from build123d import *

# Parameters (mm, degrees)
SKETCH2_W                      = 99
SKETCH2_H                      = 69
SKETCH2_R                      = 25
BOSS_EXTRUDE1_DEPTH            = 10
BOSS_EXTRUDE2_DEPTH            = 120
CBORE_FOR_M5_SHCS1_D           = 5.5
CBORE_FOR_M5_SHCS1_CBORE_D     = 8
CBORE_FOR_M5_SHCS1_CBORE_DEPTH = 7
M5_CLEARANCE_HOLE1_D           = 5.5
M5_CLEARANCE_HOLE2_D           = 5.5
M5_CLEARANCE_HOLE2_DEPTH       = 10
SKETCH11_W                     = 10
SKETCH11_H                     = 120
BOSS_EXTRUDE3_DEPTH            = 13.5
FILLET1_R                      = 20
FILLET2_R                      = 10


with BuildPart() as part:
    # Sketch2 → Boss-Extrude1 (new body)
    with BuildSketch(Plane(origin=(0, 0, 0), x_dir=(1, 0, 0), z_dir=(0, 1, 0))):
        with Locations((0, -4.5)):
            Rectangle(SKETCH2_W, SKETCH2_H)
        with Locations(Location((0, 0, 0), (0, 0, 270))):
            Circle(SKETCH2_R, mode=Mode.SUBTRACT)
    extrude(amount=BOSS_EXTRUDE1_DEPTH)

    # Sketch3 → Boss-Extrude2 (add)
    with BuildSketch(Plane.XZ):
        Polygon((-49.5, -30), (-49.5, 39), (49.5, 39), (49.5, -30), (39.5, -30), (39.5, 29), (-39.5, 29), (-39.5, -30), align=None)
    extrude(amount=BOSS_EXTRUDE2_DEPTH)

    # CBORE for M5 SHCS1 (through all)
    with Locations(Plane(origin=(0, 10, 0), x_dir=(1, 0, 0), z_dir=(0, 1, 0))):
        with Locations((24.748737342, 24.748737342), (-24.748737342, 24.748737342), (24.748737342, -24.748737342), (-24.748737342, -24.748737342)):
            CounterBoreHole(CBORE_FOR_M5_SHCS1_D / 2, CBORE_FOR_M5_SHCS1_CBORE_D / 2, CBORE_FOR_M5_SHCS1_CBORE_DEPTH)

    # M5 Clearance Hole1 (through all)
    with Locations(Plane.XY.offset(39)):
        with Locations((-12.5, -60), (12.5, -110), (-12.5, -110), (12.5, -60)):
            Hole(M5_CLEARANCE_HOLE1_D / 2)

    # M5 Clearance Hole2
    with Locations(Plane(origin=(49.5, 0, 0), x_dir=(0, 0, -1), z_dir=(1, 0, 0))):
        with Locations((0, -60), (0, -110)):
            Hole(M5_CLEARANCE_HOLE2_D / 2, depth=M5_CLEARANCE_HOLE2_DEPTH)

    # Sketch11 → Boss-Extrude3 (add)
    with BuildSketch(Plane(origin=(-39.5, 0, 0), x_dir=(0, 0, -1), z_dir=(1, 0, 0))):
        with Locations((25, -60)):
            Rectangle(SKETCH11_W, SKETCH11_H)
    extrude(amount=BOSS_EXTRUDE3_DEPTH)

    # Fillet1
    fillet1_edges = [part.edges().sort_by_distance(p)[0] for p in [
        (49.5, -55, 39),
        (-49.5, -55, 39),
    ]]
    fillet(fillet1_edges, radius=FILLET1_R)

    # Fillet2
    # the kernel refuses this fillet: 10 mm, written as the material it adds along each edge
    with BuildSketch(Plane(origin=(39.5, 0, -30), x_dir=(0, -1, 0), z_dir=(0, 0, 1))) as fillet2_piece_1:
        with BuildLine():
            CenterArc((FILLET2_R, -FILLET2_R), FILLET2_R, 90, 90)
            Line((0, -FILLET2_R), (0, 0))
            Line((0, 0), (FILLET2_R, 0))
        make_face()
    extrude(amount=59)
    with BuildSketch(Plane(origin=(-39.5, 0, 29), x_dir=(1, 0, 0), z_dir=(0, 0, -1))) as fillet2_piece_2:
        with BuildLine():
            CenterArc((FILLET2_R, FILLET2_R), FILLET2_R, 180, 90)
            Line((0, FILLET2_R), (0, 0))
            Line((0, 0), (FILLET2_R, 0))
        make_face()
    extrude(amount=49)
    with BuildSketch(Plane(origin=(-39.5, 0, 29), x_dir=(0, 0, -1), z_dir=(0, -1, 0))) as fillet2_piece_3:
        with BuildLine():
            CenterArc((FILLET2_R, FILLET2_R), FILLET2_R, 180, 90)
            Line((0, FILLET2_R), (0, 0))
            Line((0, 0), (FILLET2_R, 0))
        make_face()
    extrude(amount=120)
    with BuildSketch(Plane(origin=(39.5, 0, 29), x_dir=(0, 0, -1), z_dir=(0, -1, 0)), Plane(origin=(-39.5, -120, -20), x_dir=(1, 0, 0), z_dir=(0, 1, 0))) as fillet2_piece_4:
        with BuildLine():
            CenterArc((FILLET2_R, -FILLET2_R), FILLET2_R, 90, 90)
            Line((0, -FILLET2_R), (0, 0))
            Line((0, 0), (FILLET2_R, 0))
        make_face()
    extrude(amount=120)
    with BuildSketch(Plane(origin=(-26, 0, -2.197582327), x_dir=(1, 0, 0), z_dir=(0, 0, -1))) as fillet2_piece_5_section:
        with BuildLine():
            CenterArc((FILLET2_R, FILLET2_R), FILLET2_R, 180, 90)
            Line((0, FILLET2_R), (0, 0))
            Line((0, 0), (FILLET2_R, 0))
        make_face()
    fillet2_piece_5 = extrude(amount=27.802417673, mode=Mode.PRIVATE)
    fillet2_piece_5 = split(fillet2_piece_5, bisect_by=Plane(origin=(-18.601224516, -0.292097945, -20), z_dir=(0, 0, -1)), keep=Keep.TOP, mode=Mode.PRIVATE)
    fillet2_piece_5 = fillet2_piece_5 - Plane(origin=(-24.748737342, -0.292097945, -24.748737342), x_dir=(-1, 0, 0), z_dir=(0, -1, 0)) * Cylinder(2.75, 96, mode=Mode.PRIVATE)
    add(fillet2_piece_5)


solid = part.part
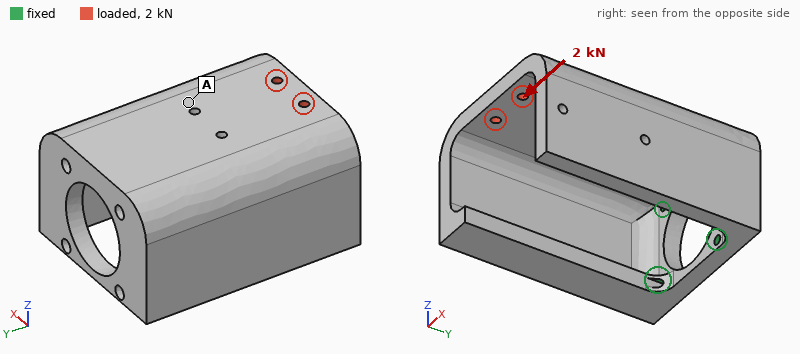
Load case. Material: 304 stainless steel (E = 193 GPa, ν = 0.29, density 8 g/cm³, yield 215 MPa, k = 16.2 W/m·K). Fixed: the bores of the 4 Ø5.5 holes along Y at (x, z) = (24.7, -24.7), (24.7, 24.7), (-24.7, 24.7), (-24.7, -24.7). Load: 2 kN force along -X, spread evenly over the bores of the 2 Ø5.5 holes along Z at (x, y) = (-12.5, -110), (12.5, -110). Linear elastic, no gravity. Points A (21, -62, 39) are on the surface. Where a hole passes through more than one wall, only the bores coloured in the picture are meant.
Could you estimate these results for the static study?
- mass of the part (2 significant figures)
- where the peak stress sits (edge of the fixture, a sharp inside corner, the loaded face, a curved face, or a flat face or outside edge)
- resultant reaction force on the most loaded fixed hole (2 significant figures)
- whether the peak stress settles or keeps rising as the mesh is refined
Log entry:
2.5 kg
edge of the fixture
4.1 kN
keeps rising
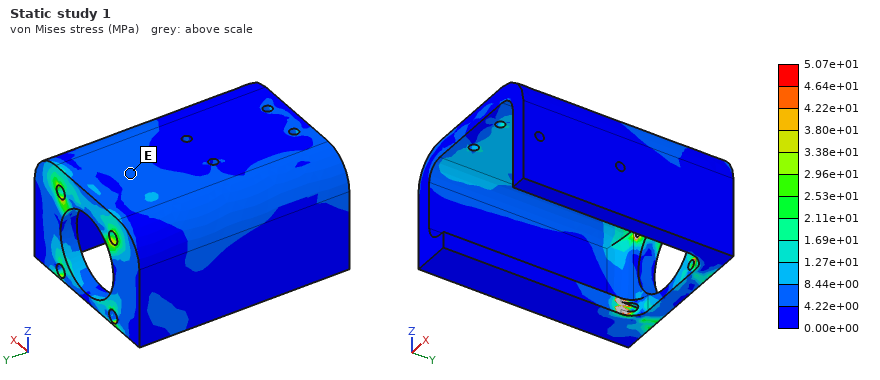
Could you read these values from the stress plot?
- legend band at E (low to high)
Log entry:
4.22e+00 to 8.44e+00 MPa
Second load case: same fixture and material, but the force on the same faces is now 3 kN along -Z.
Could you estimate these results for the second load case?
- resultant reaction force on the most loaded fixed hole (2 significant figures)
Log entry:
3.8 kN
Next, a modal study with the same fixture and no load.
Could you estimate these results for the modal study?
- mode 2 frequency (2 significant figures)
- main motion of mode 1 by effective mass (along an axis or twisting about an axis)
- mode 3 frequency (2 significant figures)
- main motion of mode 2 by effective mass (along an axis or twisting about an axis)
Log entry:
1200 Hz
along X
1700 Hz
along Z
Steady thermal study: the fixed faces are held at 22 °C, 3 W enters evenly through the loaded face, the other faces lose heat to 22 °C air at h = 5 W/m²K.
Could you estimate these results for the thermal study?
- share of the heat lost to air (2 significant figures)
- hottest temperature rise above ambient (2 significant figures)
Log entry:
48 %
15 K
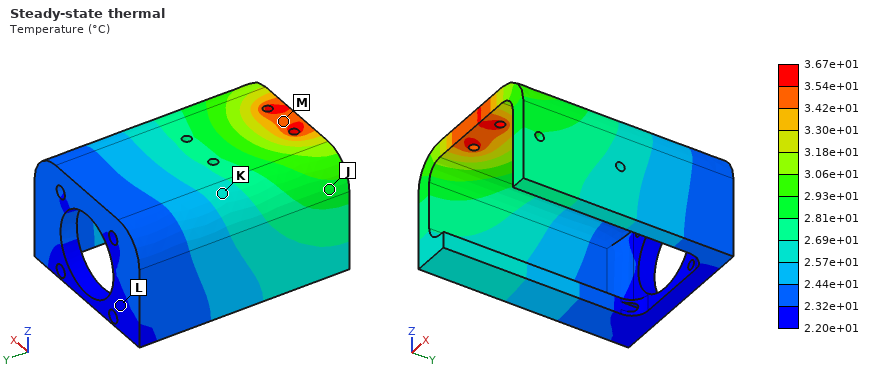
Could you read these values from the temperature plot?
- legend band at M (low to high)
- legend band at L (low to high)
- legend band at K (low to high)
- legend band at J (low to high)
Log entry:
3.42e+01 to 3.54e+01 °C
2.20e+01 to 2.32e+01 °C
2.57e+01 to 2.69e+01 °C
2.81e+01 to 2.93e+01 °C
